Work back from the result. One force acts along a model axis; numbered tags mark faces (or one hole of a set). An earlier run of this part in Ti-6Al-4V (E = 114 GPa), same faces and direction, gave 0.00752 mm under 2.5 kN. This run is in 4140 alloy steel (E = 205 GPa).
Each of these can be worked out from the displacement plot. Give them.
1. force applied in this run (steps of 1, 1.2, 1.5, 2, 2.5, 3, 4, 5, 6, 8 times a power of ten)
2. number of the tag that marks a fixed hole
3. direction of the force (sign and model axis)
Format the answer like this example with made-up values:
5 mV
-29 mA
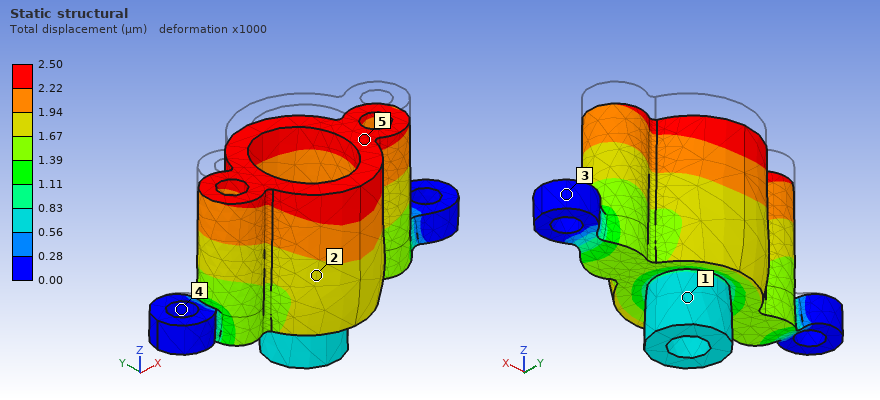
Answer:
1.5 kN
4
-Z
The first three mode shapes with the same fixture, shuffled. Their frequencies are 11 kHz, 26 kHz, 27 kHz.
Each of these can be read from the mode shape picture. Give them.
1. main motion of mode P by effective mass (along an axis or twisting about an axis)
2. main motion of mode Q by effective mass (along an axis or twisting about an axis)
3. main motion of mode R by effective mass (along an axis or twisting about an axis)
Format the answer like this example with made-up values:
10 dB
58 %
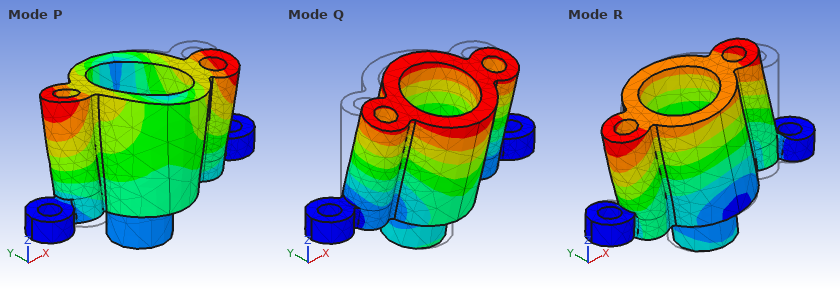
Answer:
twisting about Z
along Y
along X
